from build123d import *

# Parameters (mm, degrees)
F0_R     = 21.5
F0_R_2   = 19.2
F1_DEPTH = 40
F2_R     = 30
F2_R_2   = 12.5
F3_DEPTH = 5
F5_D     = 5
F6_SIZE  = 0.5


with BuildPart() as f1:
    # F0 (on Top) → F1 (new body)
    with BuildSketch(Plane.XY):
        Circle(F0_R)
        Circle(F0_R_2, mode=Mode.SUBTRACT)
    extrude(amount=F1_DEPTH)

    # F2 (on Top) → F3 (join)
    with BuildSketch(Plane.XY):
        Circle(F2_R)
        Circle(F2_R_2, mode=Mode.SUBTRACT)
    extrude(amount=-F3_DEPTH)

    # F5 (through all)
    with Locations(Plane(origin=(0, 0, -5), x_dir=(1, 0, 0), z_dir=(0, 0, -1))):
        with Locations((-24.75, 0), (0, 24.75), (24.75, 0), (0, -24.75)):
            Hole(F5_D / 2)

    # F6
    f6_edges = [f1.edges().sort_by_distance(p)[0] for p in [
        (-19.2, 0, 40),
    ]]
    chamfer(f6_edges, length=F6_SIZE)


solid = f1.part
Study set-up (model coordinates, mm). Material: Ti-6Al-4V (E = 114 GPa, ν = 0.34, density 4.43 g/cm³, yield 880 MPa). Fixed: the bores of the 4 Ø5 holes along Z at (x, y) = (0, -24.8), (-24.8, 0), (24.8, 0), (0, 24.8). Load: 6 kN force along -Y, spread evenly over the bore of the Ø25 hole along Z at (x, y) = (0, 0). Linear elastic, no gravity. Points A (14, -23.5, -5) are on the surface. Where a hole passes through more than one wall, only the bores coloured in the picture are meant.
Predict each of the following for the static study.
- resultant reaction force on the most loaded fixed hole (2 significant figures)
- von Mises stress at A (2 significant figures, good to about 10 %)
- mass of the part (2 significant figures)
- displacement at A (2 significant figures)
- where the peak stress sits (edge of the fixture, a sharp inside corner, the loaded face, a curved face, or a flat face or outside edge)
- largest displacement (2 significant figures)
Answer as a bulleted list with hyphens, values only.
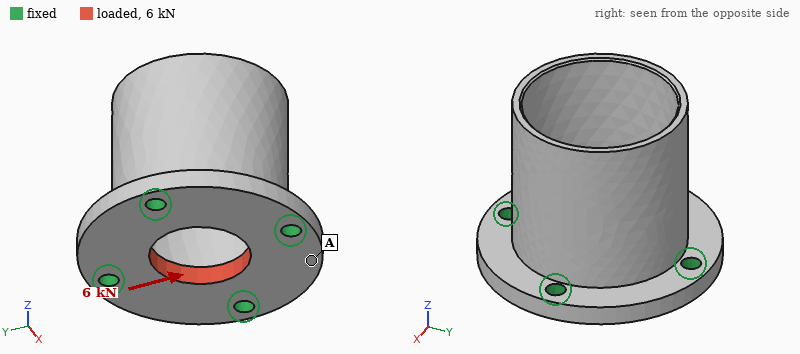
- 1.7 kN
- 7.0 MPa
- 100 g
- 2.4 µm
- edge of the fixture
- 3.9 µm
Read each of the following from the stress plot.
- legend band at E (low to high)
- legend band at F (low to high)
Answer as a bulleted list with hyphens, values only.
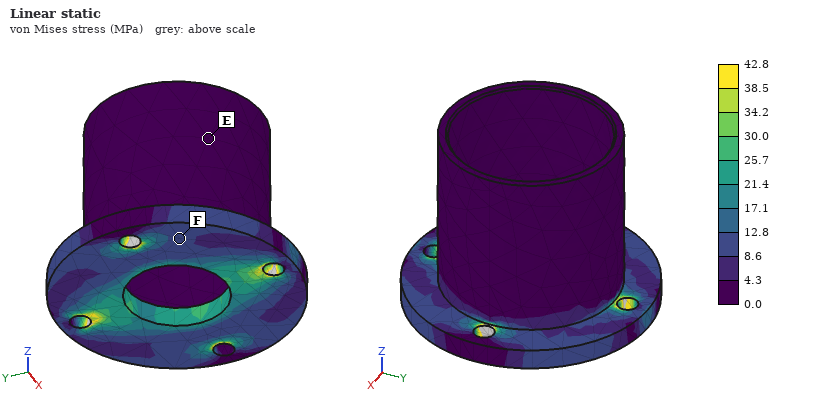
- 0.0 to 4.3 MPa
- 8.6 to 12.8 MPa
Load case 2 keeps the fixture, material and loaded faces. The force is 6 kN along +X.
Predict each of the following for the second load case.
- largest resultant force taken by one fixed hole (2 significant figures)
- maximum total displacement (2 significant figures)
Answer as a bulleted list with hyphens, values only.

- 1.7 kN
- 3.9 µm
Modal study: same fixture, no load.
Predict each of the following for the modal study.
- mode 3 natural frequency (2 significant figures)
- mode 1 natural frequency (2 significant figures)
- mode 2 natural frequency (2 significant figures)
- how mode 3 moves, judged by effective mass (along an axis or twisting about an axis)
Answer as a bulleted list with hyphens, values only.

- 8900 Hz
- 5300 Hz
- 6700 Hz
- along X
